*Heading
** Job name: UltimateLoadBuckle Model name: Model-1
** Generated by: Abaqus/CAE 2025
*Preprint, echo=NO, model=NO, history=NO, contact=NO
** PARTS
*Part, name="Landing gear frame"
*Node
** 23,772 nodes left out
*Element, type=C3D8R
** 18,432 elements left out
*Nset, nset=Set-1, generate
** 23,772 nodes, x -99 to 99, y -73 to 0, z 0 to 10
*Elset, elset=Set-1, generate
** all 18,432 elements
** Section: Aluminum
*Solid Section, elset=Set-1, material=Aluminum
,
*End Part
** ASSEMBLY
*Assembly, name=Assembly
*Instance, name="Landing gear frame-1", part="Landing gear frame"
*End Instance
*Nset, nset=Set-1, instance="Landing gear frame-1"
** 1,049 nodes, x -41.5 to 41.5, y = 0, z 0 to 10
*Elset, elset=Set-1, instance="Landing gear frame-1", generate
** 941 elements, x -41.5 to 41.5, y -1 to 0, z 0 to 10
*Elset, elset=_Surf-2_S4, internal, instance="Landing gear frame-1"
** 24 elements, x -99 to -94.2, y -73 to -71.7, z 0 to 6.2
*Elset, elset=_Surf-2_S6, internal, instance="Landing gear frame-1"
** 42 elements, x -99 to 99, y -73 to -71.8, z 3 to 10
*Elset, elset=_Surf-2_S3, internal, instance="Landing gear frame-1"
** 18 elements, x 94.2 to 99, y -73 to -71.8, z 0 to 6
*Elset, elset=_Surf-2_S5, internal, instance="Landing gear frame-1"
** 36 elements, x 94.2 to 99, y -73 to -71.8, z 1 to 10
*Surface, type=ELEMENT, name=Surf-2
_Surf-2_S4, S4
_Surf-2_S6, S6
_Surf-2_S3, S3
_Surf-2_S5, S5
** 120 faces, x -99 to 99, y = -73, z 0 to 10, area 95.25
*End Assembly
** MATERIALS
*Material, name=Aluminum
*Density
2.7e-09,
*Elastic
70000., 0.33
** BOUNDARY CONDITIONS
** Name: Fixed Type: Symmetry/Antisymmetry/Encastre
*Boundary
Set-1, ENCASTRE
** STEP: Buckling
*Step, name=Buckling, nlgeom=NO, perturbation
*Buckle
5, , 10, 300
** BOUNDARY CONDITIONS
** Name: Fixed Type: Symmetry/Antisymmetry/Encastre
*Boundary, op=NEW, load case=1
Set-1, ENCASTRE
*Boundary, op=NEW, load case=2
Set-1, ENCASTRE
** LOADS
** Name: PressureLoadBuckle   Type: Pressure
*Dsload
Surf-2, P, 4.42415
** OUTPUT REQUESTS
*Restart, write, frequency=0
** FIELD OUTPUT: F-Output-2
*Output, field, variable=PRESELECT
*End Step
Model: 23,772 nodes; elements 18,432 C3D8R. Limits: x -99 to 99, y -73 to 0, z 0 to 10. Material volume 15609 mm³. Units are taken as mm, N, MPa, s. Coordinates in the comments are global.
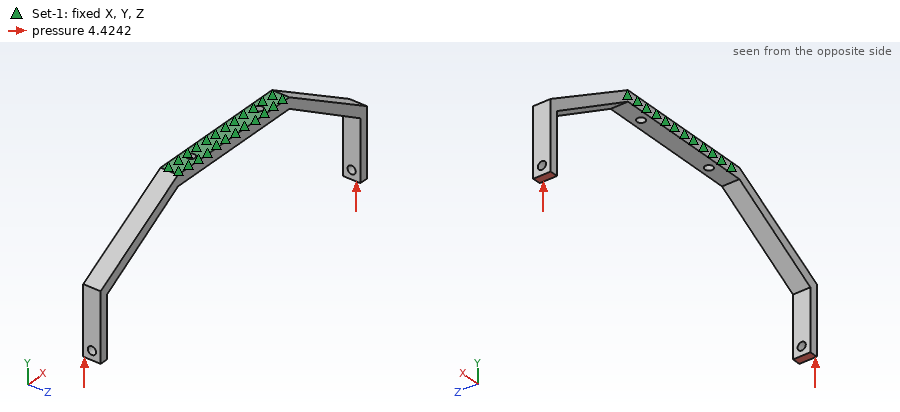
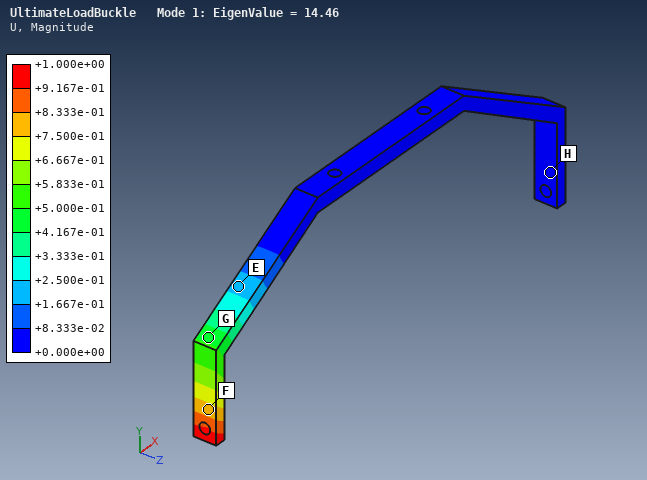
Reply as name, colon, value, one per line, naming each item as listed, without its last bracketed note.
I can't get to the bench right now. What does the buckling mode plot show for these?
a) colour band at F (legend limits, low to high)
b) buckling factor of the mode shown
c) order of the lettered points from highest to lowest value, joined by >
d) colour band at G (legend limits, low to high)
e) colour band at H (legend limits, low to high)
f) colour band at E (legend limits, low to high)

colour band at F: +7.500e-01 to +8.333e-01
buckling factor of the mode shown: 14.46
order of the lettered points from highest to lowest value, joined by >: F > G > E > H
colour band at G: +4.167e-01 to +5.000e-01
colour band at H: +0.000e+00 to +8.333e-02
colour band at E: +1.667e-01 to +2.500e-01
